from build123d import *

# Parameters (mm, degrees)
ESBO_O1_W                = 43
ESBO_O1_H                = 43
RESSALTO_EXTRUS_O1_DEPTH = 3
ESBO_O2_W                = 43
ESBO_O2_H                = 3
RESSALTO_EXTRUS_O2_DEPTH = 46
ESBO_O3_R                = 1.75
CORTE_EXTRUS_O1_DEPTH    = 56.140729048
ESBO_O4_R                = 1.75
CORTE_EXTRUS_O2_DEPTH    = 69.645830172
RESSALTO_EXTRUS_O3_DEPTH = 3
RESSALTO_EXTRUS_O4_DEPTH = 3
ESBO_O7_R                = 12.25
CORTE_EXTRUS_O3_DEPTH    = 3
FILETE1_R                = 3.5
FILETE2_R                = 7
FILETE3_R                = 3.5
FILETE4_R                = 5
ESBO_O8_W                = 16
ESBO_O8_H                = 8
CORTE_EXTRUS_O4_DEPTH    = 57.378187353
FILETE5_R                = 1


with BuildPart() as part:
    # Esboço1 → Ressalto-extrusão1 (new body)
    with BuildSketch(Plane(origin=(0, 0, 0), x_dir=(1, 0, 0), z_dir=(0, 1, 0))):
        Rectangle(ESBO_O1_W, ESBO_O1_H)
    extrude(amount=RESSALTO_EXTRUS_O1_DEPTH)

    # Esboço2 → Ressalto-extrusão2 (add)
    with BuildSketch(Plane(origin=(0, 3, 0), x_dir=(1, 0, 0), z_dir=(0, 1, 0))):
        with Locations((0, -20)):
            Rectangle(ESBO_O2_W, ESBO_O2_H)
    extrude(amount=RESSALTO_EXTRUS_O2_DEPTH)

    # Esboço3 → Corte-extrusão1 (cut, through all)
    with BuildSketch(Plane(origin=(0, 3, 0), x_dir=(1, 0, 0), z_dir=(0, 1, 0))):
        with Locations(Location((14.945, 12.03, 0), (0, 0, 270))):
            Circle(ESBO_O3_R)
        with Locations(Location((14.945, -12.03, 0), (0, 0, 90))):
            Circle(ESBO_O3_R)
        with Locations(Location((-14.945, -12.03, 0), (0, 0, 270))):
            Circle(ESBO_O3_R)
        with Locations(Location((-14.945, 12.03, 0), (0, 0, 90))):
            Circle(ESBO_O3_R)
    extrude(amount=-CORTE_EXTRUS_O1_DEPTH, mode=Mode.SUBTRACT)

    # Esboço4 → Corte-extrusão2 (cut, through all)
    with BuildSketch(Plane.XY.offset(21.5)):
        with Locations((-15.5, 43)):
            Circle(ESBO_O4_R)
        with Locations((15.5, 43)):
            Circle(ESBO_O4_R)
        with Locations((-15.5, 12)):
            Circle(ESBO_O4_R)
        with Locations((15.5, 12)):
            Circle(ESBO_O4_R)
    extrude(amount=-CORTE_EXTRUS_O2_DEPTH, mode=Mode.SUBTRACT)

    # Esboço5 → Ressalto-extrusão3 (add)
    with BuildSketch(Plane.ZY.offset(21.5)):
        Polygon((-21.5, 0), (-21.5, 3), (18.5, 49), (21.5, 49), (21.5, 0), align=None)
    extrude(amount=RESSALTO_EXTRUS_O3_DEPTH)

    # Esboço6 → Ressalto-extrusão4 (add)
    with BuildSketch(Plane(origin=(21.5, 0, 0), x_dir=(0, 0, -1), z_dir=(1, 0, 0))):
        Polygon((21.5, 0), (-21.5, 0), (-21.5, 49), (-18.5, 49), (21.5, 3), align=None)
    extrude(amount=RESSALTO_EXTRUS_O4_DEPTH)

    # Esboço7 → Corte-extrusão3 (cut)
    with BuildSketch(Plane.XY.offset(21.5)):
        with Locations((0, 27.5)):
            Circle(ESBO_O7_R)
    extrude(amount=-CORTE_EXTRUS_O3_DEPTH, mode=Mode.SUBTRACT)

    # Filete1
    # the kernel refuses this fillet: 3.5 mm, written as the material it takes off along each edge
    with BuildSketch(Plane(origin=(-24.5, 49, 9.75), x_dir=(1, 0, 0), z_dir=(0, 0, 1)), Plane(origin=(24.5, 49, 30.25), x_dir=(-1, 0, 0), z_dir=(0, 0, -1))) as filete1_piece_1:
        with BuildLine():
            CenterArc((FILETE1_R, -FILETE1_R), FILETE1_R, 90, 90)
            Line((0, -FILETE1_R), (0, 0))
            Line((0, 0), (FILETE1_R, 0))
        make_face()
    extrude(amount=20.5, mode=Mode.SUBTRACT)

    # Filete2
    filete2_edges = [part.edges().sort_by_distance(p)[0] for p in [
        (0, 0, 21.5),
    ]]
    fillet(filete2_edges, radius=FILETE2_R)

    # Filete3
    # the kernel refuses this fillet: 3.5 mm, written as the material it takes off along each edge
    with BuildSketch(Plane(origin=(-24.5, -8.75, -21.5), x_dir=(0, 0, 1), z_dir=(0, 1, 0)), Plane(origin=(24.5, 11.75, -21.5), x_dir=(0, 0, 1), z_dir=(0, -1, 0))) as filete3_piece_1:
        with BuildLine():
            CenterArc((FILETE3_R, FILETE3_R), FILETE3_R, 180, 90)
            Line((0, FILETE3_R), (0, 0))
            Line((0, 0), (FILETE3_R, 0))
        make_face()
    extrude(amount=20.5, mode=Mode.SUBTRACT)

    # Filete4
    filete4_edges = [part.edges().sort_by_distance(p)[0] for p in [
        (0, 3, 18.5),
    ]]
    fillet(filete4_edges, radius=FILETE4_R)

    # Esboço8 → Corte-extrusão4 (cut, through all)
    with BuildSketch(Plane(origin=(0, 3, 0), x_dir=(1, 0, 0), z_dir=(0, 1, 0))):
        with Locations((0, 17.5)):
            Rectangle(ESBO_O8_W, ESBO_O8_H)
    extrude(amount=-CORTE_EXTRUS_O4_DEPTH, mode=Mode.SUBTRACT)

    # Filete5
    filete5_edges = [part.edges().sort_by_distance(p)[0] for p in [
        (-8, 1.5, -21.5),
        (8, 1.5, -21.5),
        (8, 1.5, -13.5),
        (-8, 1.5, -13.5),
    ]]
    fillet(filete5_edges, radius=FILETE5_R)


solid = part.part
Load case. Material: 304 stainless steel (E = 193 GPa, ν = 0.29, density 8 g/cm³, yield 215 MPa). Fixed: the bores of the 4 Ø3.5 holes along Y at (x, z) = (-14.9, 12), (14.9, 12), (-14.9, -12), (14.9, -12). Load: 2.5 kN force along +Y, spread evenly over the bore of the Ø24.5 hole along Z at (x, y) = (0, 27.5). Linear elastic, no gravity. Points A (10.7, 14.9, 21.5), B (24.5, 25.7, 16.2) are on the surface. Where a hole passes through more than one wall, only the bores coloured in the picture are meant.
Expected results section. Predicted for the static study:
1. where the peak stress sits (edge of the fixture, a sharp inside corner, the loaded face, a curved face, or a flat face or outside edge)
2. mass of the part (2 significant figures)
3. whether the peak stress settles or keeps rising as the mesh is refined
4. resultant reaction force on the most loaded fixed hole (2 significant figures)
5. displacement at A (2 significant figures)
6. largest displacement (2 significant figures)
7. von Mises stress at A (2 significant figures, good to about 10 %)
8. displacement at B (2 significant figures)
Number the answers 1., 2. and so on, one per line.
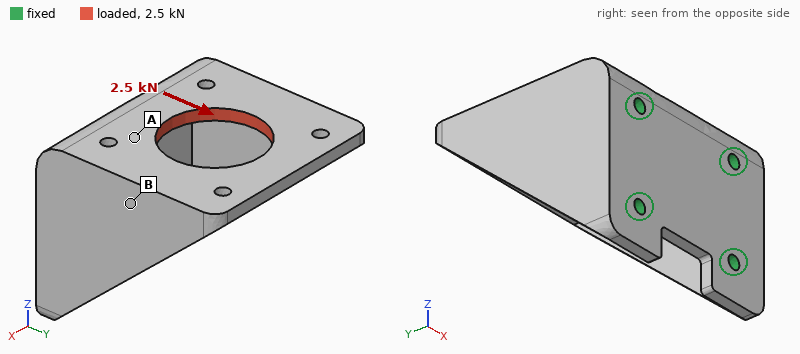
1. edge of the fixture
2. 130 g
3. keeps rising
4. 1.5 kN
5. 19 µm
6. 35 µm
7. 39 MPa
8. 16 µm
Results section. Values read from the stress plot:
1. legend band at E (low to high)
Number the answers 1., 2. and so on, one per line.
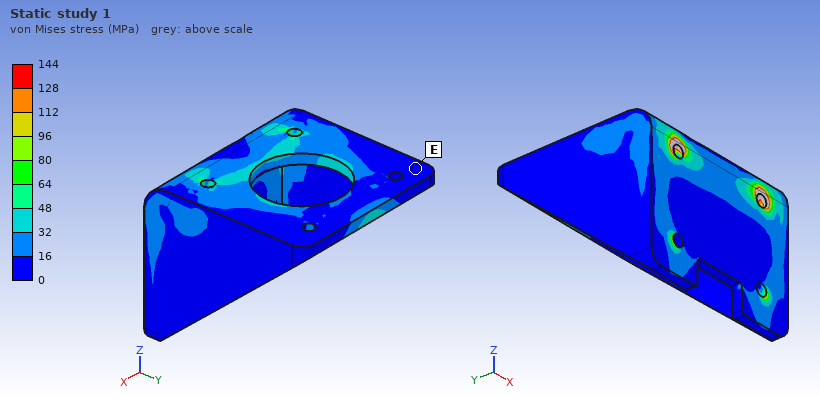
1. 0 to 16 MPa
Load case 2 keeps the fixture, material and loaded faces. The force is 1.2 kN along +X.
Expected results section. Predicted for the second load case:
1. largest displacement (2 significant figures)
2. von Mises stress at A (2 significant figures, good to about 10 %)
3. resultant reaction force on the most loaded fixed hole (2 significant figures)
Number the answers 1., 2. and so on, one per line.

1. 38 µm
2. 25 MPa
3. 1.2 kN
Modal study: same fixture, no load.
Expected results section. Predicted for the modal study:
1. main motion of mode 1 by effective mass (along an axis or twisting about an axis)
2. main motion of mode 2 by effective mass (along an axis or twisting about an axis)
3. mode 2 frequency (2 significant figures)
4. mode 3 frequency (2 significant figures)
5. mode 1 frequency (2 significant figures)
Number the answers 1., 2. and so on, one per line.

1. along Z
2. along X
3. 3800 Hz
4. 5800 Hz
5. 3400 Hz
